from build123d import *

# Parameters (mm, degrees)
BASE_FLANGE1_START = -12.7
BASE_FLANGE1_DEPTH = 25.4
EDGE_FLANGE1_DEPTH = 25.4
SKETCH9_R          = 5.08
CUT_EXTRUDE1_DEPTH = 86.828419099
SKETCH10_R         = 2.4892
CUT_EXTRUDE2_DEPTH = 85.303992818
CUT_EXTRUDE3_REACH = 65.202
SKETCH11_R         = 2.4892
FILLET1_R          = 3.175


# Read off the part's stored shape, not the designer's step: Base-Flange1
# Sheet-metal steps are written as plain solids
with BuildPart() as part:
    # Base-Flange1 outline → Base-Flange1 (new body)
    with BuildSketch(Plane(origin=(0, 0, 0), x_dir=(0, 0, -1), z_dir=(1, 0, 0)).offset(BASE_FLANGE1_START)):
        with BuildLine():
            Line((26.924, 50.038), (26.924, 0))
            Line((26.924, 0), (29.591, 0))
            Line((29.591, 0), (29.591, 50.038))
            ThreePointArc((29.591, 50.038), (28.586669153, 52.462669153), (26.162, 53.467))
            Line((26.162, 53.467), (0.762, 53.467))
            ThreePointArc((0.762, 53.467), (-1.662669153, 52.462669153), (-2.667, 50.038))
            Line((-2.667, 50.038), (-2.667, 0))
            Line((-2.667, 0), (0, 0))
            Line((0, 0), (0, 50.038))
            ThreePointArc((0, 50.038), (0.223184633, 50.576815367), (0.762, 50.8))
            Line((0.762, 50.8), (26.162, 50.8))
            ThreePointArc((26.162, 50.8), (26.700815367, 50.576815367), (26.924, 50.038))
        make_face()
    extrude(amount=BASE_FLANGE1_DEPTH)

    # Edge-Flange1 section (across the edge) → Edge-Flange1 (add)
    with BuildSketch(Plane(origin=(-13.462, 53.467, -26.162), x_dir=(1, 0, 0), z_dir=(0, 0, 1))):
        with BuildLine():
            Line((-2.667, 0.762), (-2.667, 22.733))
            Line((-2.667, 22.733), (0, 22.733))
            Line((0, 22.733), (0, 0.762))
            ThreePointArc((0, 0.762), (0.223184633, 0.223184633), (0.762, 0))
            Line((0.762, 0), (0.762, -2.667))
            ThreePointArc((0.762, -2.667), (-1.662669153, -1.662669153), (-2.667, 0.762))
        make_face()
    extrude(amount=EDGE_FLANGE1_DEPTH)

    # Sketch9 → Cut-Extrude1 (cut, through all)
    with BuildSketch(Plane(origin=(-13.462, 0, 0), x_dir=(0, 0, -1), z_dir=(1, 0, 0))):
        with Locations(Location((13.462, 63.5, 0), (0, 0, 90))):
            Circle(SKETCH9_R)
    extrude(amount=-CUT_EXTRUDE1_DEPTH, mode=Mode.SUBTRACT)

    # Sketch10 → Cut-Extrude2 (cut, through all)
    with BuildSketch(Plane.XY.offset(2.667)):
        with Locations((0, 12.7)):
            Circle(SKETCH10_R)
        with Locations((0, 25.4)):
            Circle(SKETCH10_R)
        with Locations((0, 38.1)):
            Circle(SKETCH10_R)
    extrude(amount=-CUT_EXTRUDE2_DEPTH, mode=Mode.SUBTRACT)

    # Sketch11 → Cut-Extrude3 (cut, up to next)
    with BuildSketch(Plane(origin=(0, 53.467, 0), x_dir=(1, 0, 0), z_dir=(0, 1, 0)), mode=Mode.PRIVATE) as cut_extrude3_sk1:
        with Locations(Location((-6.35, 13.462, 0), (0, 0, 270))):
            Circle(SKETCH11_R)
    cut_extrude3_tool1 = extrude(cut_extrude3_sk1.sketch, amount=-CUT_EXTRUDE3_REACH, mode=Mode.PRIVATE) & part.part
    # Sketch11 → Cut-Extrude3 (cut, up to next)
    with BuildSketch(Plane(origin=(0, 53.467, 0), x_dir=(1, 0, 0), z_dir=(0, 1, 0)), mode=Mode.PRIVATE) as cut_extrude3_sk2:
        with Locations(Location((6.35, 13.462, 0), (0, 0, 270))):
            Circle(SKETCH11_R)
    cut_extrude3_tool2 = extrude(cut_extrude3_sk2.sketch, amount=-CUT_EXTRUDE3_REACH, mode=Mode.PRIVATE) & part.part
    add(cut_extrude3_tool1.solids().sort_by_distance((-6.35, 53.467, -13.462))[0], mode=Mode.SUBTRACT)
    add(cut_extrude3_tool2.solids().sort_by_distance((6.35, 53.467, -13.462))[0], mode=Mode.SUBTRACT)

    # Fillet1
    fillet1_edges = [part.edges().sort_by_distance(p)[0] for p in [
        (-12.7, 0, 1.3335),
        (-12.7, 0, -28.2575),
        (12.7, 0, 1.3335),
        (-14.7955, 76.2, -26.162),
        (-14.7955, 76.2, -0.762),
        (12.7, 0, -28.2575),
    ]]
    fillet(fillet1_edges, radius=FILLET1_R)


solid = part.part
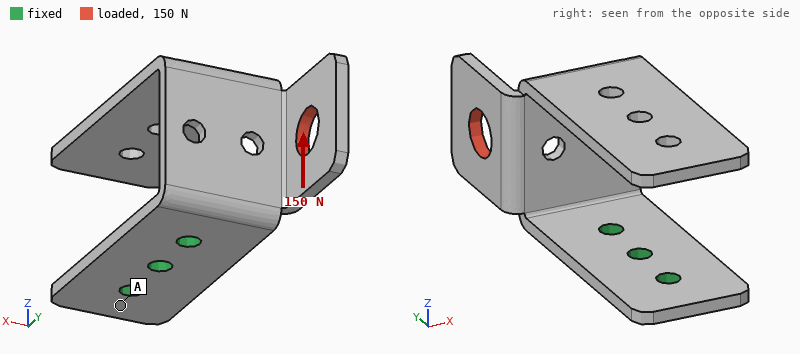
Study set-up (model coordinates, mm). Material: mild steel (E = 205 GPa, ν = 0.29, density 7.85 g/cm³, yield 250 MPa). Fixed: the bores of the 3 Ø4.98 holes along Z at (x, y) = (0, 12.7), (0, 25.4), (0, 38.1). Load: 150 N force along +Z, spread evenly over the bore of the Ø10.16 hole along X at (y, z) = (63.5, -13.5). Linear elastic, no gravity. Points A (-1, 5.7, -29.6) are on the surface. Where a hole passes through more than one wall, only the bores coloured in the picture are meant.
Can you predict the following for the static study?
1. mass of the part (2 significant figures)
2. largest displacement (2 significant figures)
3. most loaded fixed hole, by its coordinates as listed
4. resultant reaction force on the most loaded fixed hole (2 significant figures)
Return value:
78 g
0.40 mm
(0, 38.1)
230 N
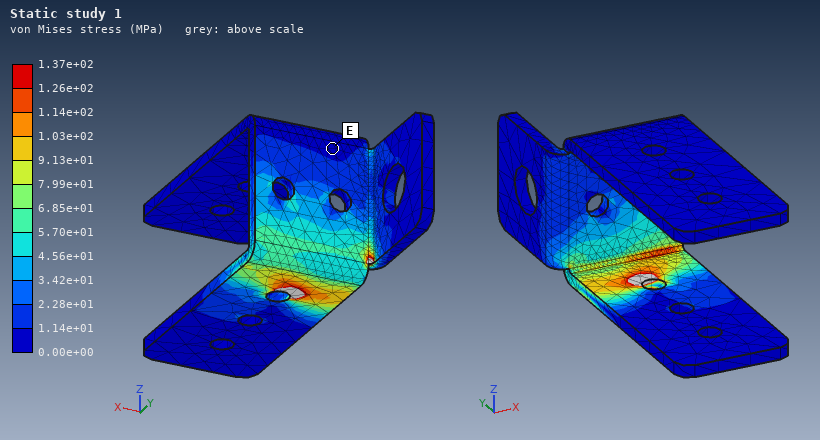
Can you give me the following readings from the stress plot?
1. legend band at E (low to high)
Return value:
0.00e+00 to 1.14e+01 MPa
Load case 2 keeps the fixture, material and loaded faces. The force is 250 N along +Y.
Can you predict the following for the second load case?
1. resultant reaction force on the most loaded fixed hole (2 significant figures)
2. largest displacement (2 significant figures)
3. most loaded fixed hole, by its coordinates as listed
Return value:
250 N
0.56 mm
(0, 38.1)
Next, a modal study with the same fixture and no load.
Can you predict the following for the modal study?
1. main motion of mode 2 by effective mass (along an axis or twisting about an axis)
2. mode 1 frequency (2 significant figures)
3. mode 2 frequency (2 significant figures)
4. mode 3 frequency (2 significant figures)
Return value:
along X
380 Hz
560 Hz
930 Hz
